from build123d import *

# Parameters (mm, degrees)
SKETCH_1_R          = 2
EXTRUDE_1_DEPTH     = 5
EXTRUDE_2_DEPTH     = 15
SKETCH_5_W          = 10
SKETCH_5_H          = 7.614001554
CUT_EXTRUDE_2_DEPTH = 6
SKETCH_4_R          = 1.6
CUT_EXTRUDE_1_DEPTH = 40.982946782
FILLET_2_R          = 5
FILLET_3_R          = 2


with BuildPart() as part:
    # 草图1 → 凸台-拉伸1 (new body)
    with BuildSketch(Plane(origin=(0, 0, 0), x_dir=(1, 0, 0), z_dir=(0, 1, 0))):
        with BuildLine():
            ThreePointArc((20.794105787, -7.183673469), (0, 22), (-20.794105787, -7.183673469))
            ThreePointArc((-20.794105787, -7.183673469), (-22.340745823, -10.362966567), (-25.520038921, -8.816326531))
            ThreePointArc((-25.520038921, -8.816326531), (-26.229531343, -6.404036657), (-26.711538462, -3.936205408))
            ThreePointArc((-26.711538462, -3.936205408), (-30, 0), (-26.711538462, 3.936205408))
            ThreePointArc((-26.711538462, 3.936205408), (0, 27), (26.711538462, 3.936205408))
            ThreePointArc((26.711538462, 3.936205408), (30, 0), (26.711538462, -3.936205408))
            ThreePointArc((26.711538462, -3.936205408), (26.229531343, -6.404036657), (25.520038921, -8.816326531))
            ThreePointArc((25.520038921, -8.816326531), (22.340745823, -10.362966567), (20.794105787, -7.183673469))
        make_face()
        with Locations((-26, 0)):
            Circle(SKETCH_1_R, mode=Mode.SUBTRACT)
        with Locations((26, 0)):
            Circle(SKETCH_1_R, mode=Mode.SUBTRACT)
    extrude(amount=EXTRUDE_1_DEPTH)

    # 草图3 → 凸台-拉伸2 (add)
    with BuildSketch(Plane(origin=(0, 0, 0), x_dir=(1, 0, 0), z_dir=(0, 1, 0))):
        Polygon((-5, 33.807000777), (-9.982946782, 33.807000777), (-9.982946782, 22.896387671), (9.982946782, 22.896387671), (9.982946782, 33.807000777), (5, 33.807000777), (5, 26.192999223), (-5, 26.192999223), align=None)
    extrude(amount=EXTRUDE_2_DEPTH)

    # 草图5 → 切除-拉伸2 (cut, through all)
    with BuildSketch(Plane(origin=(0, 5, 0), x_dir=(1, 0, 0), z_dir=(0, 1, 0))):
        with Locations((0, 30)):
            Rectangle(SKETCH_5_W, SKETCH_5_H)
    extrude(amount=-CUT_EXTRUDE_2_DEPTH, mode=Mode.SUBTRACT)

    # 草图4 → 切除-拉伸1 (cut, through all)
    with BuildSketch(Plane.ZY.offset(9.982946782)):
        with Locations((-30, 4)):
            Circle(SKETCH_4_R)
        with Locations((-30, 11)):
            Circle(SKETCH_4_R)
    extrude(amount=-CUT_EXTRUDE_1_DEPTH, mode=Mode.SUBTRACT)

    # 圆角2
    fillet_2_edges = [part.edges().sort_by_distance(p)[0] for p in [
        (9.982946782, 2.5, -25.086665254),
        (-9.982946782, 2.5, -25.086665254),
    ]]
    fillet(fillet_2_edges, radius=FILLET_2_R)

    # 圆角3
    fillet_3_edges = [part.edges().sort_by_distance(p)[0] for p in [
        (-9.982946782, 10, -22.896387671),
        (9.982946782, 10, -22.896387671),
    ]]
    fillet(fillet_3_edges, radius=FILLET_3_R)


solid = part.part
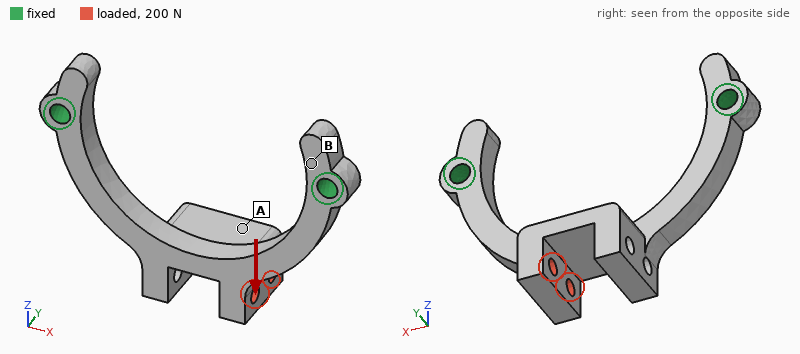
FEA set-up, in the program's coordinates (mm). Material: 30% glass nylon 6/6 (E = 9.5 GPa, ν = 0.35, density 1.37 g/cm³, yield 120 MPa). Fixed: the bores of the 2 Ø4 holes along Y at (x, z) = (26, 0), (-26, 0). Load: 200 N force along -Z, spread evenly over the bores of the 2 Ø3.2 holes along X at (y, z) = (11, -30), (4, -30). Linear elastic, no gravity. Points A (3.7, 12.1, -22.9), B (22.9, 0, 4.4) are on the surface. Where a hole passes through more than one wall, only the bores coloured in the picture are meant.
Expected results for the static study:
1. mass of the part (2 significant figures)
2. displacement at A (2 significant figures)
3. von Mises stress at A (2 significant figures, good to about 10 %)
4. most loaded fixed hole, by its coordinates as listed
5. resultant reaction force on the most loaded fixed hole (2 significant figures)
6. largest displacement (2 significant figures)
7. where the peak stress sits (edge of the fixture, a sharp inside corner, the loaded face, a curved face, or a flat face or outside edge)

5.6 g
0.51 mm
13 MPa
(26, 0)
160 N
0.89 mm
a sharp inside corner
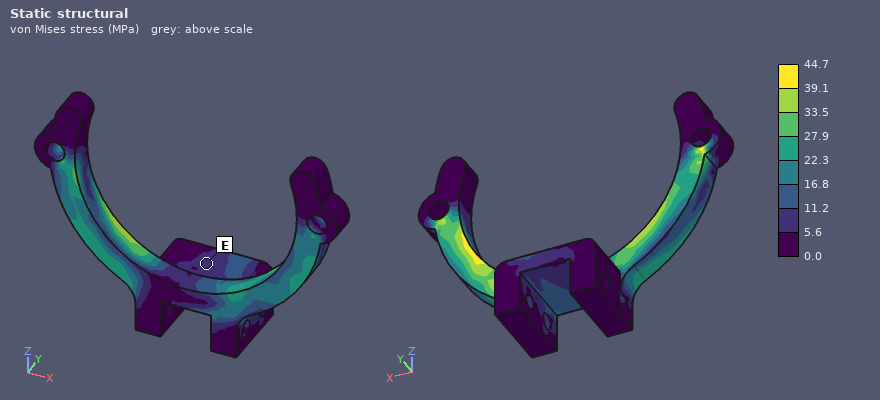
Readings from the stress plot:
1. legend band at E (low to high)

5.6 to 11.2 MPa
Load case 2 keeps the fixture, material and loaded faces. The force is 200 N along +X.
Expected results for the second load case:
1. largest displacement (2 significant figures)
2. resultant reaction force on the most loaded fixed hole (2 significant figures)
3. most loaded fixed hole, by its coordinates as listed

0.20 mm
140 N
(-26, 0)
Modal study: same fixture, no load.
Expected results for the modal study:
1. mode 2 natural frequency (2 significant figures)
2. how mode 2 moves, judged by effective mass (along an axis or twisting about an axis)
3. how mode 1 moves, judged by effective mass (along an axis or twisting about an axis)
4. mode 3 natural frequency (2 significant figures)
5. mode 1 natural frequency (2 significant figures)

2900 Hz
along X
along Y
3500 Hz
950 Hz
